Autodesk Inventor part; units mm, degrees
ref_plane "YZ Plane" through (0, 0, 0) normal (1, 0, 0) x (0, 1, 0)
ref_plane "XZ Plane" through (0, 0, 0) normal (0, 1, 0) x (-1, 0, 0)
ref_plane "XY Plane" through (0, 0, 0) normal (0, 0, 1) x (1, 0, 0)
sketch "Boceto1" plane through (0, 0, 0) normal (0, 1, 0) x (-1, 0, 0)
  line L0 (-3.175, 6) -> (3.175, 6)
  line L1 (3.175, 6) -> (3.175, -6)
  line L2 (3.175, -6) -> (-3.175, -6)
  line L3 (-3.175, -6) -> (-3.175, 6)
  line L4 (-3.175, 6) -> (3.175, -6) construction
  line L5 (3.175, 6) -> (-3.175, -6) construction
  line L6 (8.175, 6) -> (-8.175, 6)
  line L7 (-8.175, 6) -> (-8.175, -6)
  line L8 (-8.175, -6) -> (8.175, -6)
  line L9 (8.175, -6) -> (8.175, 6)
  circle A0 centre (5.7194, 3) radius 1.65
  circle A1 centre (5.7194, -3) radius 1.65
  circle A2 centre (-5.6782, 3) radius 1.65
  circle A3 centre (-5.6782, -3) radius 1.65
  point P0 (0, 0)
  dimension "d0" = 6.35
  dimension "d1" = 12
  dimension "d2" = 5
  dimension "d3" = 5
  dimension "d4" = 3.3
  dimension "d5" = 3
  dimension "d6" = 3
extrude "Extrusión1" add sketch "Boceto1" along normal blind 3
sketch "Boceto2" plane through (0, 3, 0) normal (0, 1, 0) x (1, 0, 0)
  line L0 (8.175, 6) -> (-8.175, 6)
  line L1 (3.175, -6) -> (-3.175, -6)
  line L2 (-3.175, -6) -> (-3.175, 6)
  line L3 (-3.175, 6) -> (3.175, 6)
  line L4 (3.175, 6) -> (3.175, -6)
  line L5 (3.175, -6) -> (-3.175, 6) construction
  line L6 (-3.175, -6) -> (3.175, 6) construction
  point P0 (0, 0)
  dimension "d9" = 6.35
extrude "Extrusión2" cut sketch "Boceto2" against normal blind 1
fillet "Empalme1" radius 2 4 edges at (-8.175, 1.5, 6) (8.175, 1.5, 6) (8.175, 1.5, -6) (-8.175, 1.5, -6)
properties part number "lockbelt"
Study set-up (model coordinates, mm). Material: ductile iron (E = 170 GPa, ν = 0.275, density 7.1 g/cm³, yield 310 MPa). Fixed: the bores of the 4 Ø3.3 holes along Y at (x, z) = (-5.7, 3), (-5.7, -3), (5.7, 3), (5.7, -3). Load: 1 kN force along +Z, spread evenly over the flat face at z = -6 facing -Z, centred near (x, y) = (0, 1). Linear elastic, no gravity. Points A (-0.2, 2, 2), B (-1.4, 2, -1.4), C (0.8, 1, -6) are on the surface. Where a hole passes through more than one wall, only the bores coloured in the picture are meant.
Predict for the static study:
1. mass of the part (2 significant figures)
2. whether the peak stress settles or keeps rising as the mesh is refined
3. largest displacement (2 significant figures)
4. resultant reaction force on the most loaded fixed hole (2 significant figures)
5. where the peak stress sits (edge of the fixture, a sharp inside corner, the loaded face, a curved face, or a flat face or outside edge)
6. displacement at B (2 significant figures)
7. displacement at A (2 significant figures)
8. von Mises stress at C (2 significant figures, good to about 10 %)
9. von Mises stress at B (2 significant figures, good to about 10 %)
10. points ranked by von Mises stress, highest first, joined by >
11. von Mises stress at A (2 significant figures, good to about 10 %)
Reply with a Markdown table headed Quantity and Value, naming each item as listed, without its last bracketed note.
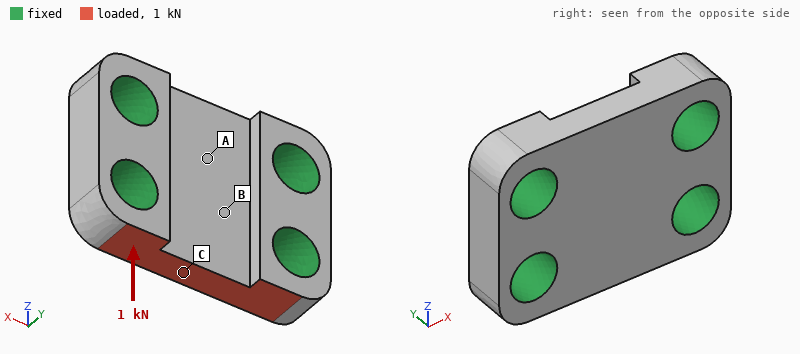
| Quantity | Value |
|---|---|
| mass of the part | 2.8 g |
| whether the peak stress settles or keeps rising as the mesh is refined | keeps rising |
| largest displacement | 1.2 µm |
| resultant reaction force on the most loaded fixed hole | 420 N |
| where the peak stress sits | edge of the fixture |
| displacement at B | 0.45 µm |
| displacement at A | 0.27 µm |
| von Mises stress at C | 32 MPa |
| von Mises stress at B | 18 MPa |
| points ranked by von Mises stress, highest first, joined by > | C > B > A |
| von Mises stress at A | 6.3 MPa |
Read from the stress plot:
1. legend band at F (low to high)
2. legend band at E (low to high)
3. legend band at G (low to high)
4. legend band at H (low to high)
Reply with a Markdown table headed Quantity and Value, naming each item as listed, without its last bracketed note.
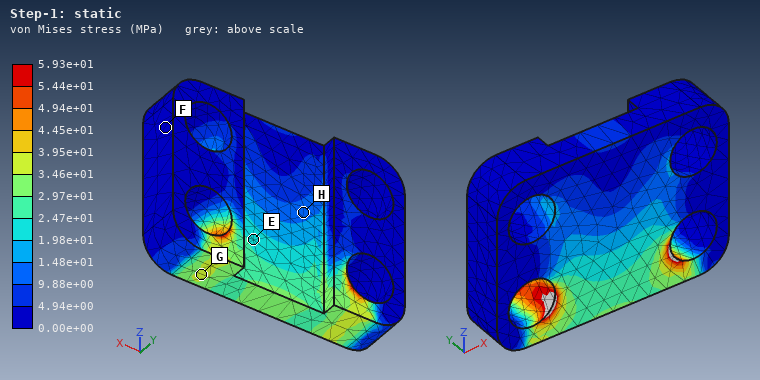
| Quantity | Value |
|---|---|
| legend band at F | 0.00e+00 to 4.94e+00 MPa |
| legend band at E | 1.98e+01 to 2.47e+01 MPa |
| legend band at G | 3.46e+01 to 3.95e+01 MPa |
| legend band at H | 9.88e+00 to 1.48e+01 MPa |
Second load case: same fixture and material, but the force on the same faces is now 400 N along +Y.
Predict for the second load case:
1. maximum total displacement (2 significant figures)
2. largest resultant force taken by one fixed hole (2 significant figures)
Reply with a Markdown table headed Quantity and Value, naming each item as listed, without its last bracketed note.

| Quantity | Value |
|---|---|
| maximum total displacement | 3.2 µm |
| largest resultant force taken by one fixed hole | 210 N |
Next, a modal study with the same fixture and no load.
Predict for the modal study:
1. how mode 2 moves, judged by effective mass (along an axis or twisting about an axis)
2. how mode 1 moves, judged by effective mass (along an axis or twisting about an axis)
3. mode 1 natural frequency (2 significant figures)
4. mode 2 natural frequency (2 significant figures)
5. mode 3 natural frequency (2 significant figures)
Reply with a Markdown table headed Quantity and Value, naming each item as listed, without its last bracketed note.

| Quantity | Value |
|---|---|
| how mode 2 moves, judged by effective mass | twisting about X |
| how mode 1 moves, judged by effective mass | along Y |
| mode 1 natural frequency | 110 kHz |
| mode 2 natural frequency | 120 kHz |
| mode 3 natural frequency | 150 kHz |
